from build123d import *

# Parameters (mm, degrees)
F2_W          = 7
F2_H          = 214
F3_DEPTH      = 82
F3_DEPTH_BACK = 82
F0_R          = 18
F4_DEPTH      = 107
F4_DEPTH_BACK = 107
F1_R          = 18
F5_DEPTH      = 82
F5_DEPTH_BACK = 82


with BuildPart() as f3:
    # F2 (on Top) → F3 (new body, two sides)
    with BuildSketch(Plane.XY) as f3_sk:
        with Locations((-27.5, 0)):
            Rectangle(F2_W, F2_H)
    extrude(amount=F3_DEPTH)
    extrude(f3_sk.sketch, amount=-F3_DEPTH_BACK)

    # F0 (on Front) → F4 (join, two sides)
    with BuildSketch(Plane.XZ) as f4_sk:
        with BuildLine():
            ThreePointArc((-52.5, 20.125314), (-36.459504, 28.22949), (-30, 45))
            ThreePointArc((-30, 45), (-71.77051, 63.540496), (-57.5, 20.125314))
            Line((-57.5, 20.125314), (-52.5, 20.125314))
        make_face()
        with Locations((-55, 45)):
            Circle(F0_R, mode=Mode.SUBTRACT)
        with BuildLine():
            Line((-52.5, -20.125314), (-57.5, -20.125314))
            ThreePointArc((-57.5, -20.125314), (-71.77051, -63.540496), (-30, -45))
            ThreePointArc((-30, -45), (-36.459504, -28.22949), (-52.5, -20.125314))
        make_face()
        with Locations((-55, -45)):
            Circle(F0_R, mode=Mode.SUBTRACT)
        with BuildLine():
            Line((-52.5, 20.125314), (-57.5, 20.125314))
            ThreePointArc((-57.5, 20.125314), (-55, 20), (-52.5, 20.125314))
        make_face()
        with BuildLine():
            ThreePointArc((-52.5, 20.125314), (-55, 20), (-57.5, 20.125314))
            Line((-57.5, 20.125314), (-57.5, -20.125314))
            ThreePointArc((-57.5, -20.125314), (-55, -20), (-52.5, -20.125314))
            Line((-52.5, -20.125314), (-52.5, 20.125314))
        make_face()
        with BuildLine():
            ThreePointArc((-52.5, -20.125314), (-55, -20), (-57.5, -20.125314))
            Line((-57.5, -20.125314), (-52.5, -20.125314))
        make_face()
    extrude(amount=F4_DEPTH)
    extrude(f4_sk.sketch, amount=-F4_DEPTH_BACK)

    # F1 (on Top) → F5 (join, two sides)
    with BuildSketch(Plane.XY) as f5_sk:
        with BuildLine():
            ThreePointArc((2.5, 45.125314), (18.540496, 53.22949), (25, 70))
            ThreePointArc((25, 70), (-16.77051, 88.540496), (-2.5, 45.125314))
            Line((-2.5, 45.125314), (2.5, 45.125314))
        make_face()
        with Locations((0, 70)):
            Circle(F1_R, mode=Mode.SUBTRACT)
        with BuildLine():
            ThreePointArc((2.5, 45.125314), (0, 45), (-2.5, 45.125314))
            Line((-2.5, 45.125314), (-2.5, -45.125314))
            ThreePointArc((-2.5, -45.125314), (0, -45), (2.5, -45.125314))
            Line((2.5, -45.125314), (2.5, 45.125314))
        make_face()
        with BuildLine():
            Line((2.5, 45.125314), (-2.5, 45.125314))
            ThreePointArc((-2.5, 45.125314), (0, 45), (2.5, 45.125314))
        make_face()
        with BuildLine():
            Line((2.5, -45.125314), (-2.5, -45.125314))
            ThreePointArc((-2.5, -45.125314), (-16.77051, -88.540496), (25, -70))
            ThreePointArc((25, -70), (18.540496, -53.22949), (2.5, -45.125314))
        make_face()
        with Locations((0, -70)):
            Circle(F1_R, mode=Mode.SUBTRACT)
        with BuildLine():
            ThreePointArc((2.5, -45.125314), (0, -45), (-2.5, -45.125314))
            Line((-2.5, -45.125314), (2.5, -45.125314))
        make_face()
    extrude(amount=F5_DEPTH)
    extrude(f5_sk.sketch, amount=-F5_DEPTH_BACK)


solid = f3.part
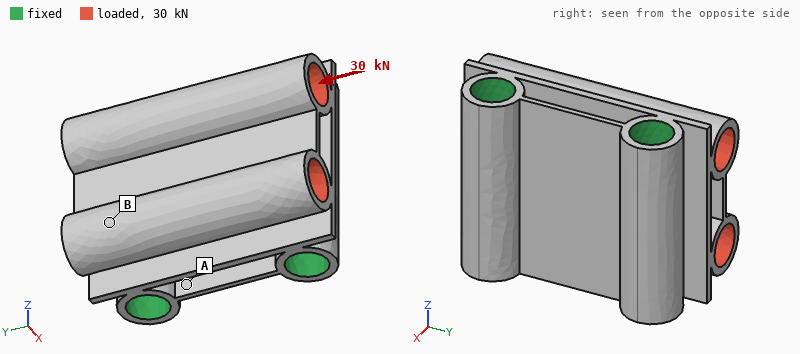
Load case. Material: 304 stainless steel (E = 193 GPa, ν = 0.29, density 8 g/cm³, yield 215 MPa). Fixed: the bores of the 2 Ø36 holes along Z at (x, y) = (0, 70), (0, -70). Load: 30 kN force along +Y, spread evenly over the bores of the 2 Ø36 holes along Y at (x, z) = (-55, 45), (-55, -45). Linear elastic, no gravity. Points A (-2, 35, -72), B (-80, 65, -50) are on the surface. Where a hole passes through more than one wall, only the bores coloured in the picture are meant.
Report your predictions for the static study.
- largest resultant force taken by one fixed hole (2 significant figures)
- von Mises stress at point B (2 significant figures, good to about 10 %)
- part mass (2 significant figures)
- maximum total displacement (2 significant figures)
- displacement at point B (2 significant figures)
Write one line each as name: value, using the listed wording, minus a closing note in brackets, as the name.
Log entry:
largest resultant force taken by one fixed hole: 16 kN
von Mises stress at point B: 4.4 MPa
part mass: 8.6 kg
maximum total displacement: 9.6 µm
displacement at point B: 7.6 µm
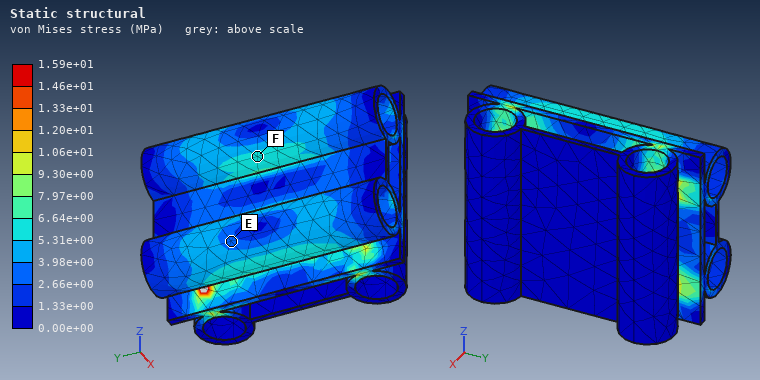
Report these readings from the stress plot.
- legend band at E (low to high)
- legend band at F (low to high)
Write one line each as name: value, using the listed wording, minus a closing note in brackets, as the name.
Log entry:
legend band at E: 2.66e+00 to 3.98e+00 MPa
legend band at F: 5.31e+00 to 6.64e+00 MPa
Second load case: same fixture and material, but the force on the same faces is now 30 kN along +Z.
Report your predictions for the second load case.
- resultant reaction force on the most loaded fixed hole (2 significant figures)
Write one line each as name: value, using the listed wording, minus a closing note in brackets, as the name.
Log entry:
resultant reaction force on the most loaded fixed hole: 15 kN
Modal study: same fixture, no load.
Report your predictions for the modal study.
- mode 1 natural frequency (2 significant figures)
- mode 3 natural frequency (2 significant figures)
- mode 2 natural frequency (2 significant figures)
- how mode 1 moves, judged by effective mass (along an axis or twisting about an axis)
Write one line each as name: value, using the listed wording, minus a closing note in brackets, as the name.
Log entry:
mode 1 natural frequency: 2400 Hz
mode 3 natural frequency: 3200 Hz
mode 2 natural frequency: 3000 Hz
how mode 1 moves, judged by effective mass: along Z
